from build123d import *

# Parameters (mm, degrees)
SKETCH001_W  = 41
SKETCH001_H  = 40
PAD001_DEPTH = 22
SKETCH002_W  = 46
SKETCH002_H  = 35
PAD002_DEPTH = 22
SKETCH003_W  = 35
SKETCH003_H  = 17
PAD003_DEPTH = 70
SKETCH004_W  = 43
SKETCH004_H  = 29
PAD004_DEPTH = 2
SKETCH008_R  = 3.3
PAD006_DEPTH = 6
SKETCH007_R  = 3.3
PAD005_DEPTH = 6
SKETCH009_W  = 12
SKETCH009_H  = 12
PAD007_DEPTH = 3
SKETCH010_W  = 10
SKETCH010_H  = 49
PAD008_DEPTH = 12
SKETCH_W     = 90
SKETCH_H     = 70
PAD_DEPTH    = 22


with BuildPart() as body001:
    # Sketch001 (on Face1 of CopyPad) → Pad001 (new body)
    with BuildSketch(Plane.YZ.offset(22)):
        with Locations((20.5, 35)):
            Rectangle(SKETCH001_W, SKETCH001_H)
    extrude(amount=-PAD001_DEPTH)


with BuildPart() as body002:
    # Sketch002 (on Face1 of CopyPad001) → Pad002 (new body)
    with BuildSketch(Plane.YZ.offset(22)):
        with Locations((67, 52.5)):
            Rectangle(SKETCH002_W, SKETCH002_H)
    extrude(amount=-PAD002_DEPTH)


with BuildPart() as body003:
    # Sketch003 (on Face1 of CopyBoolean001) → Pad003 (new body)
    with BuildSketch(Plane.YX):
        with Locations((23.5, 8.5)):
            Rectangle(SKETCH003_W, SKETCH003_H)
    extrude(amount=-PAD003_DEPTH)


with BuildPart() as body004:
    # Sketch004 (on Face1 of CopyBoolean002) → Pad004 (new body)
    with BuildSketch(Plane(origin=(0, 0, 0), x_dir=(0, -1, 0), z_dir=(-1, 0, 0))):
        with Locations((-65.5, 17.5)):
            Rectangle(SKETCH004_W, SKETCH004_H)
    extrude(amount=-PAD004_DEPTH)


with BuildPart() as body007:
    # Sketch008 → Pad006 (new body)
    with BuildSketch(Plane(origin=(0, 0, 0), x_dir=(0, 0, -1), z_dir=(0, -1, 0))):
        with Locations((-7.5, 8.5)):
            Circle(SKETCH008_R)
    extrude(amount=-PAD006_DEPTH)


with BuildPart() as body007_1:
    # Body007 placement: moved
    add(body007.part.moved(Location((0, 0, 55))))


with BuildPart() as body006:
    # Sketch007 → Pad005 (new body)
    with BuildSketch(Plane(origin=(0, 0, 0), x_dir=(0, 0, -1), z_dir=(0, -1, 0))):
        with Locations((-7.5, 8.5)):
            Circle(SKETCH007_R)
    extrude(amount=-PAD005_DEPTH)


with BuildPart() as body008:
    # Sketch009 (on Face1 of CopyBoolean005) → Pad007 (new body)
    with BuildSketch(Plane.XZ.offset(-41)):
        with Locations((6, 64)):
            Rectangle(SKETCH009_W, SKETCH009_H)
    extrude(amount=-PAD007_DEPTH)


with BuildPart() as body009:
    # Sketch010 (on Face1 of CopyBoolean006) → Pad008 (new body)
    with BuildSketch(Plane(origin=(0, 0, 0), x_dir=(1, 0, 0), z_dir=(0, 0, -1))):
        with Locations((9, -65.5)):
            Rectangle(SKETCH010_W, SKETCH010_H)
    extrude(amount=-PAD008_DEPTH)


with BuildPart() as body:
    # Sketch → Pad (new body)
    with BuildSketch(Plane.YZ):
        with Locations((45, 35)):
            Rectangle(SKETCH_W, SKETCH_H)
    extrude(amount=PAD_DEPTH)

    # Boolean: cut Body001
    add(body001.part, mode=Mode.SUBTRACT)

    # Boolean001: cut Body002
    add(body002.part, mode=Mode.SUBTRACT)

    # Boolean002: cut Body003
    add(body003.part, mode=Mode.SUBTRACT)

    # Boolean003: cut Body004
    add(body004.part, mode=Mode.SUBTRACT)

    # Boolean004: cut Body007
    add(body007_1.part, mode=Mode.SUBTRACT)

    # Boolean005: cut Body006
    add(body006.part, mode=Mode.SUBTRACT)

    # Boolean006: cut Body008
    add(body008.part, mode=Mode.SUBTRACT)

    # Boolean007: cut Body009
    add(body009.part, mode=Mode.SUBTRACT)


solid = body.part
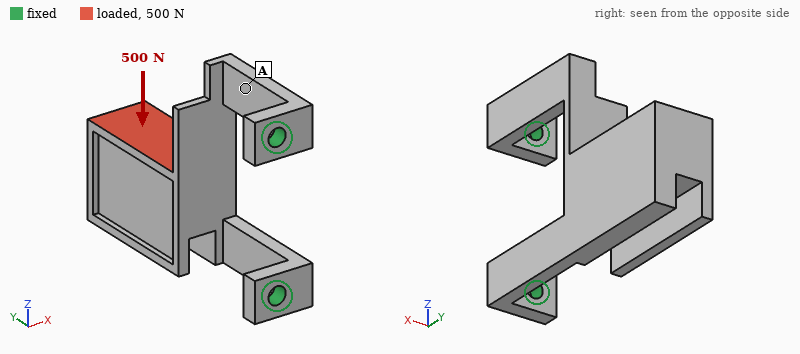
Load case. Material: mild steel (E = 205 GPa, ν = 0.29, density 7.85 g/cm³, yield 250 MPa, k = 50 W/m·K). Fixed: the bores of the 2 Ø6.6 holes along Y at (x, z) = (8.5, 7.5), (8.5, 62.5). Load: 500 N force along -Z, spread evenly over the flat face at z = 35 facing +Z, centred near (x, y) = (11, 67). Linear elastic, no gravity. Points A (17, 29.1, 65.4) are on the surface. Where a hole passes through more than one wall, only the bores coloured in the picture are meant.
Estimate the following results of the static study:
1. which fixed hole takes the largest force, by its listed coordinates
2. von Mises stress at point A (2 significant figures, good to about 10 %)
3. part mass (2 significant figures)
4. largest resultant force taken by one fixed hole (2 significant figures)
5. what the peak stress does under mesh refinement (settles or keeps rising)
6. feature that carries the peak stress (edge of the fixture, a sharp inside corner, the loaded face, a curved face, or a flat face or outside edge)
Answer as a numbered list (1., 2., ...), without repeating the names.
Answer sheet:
1. (8.5, 62.5)
2. 21 MPa
3. 310 g
4. 450 N
5. keeps rising
6. a sharp inside corner
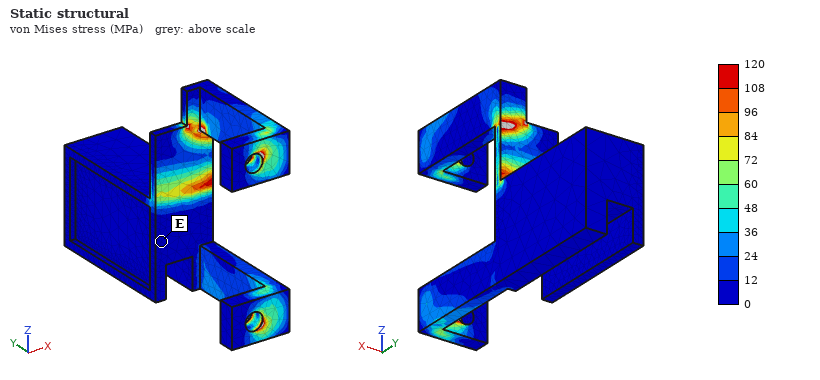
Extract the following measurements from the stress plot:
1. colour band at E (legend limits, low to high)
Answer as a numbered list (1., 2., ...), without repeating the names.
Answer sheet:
1. 0 to 12 MPa
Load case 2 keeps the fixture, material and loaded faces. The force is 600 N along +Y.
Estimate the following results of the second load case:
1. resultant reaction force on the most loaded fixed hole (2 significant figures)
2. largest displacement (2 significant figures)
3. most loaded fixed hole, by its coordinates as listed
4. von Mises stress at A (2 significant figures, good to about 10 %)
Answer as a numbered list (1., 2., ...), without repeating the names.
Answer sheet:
1. 390 N
2. 0.29 mm
3. (8.5, 7.5)
4. 31 MPa
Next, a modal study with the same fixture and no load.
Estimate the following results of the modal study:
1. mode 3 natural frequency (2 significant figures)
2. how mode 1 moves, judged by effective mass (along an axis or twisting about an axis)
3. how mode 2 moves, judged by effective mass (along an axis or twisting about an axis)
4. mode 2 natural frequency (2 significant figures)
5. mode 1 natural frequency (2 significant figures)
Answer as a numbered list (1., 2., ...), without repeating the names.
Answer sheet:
1. 1500 Hz
2. along X
3. along Z
4. 810 Hz
5. 240 Hz
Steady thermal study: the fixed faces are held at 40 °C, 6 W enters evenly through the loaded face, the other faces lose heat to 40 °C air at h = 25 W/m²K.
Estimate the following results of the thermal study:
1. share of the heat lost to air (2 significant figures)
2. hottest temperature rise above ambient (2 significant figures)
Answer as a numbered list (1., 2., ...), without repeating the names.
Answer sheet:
1. 70 %
2. 21 K
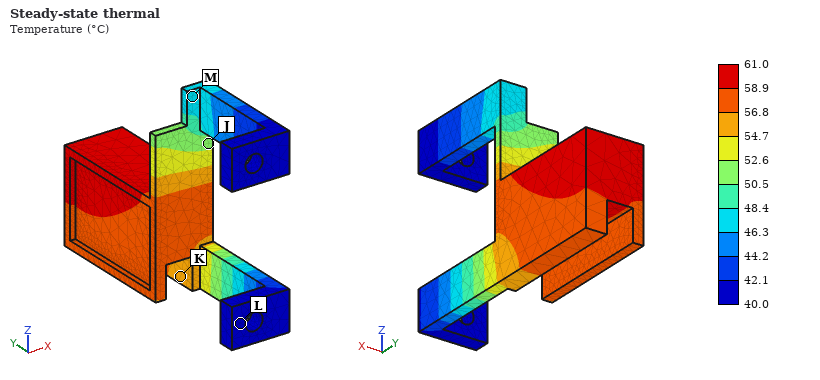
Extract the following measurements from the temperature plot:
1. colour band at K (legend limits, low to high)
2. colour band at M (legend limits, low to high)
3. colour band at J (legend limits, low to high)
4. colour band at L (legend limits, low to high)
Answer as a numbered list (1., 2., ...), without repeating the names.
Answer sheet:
1. 54.7 to 56.8 °C
2. 46.3 to 48.4 °C
3. 50.5 to 52.6 °C
4. 40.0 to 42.1 °C
